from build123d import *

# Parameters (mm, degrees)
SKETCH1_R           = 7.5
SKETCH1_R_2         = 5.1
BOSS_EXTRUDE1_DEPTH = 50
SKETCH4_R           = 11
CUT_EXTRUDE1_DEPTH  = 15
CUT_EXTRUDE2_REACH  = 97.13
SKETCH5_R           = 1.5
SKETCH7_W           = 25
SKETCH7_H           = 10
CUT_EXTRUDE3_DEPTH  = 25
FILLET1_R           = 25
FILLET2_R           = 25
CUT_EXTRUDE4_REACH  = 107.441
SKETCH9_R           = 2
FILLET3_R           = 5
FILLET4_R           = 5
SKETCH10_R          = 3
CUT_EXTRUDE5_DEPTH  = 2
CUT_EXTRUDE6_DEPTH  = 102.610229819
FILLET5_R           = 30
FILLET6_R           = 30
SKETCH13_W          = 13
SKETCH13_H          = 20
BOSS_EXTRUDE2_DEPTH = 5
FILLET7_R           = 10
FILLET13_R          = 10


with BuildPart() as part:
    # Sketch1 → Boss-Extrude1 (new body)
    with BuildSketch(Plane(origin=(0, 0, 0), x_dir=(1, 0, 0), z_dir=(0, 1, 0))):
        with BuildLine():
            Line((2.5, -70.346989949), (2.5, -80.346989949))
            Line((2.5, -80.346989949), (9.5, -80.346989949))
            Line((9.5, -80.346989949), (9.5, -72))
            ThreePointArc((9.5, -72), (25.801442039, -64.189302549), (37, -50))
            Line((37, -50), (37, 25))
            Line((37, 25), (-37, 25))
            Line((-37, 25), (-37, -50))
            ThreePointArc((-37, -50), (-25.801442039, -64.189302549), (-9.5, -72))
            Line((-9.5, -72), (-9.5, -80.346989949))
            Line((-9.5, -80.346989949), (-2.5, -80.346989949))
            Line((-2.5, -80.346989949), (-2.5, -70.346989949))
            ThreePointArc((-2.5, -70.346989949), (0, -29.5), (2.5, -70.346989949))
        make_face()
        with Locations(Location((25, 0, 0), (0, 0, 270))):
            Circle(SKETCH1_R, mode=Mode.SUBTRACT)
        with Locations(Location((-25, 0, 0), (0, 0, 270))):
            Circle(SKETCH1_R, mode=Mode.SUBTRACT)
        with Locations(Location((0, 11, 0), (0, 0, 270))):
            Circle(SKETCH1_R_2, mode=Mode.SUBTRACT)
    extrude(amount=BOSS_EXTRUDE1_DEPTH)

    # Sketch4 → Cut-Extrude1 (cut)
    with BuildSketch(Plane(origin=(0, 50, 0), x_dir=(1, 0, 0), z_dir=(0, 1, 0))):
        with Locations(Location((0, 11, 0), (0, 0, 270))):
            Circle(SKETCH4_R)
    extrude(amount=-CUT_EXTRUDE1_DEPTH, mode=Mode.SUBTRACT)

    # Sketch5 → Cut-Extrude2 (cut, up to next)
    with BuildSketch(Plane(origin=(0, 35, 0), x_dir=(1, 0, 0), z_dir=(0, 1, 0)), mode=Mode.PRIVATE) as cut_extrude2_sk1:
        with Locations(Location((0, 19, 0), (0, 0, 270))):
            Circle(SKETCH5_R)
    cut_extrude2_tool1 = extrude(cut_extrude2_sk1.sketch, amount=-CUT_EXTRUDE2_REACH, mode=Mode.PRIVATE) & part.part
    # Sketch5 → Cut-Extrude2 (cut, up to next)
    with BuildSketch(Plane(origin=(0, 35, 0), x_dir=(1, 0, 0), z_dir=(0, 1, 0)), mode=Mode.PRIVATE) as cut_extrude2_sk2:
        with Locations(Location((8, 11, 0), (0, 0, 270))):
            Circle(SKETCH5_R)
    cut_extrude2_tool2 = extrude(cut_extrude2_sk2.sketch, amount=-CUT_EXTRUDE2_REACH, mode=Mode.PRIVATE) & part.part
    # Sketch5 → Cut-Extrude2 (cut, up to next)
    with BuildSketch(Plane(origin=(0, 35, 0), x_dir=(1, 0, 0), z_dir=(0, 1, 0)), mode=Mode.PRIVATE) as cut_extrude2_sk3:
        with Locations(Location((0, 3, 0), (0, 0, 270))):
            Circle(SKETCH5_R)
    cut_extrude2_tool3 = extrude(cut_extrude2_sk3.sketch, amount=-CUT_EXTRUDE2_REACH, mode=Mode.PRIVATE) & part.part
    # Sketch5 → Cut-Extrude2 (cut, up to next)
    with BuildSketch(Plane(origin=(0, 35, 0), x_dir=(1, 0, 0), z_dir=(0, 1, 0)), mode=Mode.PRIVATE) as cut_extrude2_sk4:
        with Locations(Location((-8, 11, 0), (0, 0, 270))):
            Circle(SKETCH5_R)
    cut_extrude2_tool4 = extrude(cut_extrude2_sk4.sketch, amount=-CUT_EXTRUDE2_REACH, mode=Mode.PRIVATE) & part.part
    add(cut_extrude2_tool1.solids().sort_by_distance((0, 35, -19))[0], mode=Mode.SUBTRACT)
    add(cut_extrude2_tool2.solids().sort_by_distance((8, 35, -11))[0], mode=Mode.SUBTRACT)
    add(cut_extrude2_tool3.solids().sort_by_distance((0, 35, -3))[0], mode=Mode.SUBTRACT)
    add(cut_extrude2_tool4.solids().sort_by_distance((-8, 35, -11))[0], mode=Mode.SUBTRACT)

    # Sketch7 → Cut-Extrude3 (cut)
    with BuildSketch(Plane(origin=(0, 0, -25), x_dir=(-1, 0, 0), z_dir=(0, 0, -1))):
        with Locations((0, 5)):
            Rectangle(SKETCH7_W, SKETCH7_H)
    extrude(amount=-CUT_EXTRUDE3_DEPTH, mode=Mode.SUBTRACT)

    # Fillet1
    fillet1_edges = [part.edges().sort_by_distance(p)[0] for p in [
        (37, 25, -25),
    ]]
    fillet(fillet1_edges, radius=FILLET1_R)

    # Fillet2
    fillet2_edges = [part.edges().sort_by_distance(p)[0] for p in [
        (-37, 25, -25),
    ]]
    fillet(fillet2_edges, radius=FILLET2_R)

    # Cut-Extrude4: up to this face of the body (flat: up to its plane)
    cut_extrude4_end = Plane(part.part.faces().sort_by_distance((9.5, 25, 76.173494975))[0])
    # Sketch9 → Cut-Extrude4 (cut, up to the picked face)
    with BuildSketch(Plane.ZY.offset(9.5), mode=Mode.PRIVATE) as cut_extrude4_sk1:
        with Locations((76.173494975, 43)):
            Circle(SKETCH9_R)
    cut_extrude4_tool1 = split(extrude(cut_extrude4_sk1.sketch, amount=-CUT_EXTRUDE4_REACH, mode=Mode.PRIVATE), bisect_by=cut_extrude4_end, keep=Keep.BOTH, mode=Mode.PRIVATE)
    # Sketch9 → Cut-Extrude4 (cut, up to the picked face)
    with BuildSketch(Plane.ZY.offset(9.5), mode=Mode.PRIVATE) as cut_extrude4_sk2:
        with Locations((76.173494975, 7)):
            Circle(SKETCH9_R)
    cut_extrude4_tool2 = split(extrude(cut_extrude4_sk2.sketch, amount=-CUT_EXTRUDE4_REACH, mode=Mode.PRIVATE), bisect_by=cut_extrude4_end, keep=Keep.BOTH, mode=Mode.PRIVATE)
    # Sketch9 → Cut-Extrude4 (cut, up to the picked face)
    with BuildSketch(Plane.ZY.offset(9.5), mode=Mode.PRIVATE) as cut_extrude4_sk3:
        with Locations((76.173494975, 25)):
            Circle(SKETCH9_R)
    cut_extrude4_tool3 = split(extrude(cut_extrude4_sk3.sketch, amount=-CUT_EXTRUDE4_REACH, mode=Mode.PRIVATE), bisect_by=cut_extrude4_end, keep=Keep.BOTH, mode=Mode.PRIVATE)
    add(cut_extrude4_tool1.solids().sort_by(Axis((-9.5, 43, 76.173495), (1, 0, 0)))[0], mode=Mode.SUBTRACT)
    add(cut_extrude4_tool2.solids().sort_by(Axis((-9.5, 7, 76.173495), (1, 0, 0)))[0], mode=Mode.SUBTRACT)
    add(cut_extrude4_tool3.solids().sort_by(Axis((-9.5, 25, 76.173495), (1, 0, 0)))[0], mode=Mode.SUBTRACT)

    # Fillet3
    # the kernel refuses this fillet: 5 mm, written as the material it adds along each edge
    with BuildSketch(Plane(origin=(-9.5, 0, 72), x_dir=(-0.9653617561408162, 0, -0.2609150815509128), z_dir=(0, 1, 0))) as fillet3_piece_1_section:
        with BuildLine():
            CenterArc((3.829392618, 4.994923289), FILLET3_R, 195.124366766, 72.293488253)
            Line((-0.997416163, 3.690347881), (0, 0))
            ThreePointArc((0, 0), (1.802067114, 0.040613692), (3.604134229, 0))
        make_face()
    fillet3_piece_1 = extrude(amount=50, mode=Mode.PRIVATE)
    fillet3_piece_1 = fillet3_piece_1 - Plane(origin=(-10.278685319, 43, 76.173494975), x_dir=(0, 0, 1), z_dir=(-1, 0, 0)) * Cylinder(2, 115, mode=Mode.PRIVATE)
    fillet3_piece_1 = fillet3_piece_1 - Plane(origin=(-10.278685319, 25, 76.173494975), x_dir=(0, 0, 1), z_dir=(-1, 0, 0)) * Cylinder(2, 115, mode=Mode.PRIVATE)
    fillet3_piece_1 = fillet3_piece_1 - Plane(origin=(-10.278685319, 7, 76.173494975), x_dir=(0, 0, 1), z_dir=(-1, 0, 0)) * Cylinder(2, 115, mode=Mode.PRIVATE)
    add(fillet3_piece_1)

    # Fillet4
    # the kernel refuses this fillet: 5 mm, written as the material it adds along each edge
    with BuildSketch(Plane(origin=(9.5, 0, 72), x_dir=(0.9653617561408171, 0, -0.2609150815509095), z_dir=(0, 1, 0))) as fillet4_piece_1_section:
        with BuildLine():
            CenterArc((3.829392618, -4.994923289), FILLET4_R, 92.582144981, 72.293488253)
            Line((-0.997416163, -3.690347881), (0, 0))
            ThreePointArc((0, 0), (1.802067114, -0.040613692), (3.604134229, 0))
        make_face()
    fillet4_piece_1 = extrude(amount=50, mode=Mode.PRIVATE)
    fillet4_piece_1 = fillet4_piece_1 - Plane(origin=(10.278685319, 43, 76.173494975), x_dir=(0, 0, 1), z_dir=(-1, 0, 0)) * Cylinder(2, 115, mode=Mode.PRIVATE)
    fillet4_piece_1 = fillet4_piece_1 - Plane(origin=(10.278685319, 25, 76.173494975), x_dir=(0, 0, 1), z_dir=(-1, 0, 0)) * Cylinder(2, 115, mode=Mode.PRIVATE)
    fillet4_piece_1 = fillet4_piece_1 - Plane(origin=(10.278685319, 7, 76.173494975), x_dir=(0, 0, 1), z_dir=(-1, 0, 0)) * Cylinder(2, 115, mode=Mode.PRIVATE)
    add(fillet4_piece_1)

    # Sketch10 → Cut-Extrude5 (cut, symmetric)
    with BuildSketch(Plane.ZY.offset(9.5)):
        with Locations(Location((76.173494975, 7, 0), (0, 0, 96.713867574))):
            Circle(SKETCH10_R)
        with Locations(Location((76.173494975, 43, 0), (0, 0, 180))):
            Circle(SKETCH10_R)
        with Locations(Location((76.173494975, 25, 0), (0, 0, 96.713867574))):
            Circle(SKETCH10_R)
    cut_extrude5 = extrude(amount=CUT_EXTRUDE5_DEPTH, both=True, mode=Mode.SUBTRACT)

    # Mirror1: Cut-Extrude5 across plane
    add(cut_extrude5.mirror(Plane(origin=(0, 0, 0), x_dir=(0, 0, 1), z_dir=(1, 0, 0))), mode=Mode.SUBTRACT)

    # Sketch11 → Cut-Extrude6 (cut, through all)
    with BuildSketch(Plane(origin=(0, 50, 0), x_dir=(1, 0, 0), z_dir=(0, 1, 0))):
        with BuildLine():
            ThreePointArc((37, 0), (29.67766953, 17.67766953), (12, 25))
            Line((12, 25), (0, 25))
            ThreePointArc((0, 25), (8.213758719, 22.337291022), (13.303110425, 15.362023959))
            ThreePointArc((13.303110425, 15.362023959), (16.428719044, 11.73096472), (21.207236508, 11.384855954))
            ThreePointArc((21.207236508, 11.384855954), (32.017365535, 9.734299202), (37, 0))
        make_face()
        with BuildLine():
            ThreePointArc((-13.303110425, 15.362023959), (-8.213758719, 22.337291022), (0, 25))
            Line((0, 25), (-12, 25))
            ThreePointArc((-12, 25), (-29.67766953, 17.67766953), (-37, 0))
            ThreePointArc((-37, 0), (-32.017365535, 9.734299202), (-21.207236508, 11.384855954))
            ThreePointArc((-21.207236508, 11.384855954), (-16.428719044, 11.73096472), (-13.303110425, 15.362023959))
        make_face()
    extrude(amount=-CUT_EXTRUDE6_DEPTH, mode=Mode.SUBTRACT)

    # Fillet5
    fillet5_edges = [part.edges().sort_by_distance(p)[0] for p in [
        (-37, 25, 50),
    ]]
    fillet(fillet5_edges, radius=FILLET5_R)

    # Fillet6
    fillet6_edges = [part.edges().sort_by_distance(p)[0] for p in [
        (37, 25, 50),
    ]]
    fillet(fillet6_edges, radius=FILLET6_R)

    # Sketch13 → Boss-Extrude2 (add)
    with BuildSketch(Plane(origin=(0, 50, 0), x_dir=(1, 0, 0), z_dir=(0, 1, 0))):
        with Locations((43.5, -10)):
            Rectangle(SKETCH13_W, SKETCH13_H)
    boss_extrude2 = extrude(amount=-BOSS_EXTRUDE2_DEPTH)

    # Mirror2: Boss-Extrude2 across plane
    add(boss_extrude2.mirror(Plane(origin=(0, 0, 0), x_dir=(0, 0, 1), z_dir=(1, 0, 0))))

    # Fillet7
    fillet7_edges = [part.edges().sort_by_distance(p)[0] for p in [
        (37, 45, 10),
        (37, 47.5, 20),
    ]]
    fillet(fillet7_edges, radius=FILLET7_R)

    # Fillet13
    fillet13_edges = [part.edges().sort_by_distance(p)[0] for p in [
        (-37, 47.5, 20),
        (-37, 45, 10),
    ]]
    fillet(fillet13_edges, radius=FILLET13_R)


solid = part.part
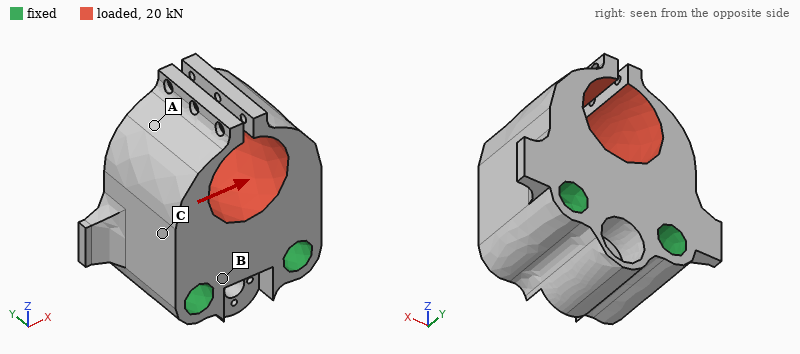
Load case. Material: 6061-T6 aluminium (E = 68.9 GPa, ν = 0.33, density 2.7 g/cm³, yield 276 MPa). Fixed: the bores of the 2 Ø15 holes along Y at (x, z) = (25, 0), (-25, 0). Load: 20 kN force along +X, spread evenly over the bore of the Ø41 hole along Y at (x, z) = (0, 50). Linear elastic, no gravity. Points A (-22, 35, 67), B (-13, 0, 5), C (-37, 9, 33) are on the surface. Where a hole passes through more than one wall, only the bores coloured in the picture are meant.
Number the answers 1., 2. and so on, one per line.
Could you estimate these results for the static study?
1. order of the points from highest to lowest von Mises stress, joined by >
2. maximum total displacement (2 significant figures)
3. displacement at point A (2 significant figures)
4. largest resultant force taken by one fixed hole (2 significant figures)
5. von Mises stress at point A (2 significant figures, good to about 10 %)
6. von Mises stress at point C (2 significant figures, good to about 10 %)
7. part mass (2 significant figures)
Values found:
1. C > A > B
2. 0.14 mm
3. 0.082 mm
4. 18 kN
5. 20 MPa
6. 34 MPa
7. 570 g
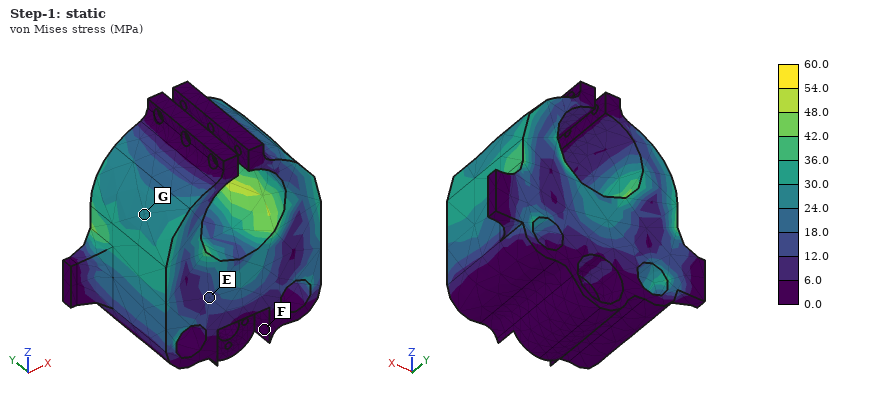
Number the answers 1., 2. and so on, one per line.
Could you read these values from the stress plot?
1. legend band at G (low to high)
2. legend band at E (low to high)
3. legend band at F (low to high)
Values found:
1. 24.0 to 30.0 MPa
2. 12.0 to 18.0 MPa
3. 0.0 to 6.0 MPa
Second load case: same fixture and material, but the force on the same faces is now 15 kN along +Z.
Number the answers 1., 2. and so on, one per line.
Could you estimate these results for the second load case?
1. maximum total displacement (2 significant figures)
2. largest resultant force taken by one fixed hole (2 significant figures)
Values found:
1. 0.13 mm
2. 8.1 kN
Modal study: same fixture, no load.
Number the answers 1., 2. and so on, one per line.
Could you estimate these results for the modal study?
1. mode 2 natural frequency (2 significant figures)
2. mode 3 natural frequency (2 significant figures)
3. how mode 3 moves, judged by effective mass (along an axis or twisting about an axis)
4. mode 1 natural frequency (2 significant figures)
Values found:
1. 4800 Hz
2. 7300 Hz
3. along Y
4. 4800 Hz
